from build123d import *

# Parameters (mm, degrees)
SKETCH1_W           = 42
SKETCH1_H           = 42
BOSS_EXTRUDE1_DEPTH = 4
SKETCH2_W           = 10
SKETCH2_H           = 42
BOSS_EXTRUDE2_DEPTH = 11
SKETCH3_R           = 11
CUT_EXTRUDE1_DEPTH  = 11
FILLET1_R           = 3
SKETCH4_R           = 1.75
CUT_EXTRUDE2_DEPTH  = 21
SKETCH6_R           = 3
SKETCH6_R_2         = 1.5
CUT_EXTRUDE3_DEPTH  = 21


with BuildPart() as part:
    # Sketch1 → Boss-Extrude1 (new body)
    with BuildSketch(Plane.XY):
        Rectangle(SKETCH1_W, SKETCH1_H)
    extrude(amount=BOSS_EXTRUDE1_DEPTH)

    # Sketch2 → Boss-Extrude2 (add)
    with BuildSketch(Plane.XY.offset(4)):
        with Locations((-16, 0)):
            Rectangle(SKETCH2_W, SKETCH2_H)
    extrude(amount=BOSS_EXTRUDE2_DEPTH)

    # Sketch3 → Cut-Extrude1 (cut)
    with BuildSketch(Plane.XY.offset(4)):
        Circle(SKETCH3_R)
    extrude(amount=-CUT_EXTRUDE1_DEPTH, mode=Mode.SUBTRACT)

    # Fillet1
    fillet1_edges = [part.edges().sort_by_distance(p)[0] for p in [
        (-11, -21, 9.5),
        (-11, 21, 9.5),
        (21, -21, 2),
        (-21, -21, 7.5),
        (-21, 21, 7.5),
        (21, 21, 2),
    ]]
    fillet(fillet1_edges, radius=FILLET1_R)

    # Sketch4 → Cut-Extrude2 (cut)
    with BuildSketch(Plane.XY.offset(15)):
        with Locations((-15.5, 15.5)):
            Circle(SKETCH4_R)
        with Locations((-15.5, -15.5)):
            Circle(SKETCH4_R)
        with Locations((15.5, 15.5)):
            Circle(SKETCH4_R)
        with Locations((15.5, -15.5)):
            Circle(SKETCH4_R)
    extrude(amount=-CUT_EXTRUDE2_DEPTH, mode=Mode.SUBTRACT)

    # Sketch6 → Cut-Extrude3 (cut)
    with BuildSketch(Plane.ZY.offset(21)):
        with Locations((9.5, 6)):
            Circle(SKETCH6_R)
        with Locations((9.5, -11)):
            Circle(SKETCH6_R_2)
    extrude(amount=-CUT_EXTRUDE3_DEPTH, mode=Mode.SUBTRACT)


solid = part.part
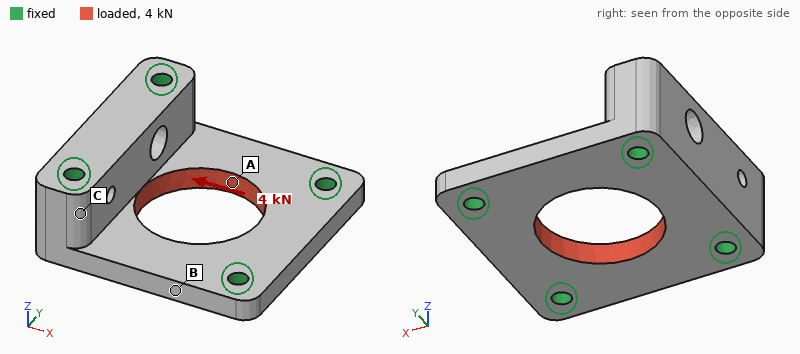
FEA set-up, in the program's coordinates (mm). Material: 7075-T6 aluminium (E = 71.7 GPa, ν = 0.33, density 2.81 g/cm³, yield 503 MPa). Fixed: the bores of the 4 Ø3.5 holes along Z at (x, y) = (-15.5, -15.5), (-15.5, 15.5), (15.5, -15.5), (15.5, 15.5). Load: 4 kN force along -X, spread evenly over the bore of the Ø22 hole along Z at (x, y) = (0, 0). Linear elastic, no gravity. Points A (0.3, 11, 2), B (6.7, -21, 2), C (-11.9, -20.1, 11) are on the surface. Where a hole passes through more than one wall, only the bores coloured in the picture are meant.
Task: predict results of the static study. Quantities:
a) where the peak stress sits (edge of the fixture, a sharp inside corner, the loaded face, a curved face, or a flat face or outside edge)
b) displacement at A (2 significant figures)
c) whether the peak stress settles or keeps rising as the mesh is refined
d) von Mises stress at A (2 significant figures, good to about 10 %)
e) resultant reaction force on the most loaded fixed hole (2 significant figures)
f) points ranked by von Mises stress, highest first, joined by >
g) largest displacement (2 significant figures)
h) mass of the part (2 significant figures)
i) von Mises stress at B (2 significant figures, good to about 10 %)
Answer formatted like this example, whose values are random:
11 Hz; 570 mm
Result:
edge of the fixture; 3.9 µm; keeps rising; 26 MPa; 1.1 kN; A > B > C; 9.3 µm; 26 g; 12 MPa
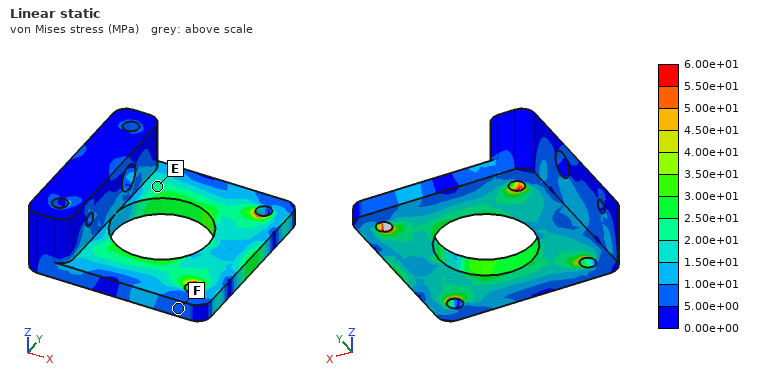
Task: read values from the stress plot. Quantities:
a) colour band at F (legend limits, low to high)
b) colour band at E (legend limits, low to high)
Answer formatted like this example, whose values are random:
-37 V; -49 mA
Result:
5.00e+00 to 1.00e+01 MPa; 2.00e+01 to 2.50e+01 MPa
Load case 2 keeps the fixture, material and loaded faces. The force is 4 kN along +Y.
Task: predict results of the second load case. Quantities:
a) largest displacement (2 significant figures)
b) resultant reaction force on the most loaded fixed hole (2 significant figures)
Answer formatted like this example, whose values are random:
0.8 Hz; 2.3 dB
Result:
8.0 µm; 1.1 kN
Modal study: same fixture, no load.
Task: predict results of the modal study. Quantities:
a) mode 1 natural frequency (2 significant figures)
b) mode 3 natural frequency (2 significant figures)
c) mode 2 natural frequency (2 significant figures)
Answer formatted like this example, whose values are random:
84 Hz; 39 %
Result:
21 kHz; 25 kHz; 24 kHz
